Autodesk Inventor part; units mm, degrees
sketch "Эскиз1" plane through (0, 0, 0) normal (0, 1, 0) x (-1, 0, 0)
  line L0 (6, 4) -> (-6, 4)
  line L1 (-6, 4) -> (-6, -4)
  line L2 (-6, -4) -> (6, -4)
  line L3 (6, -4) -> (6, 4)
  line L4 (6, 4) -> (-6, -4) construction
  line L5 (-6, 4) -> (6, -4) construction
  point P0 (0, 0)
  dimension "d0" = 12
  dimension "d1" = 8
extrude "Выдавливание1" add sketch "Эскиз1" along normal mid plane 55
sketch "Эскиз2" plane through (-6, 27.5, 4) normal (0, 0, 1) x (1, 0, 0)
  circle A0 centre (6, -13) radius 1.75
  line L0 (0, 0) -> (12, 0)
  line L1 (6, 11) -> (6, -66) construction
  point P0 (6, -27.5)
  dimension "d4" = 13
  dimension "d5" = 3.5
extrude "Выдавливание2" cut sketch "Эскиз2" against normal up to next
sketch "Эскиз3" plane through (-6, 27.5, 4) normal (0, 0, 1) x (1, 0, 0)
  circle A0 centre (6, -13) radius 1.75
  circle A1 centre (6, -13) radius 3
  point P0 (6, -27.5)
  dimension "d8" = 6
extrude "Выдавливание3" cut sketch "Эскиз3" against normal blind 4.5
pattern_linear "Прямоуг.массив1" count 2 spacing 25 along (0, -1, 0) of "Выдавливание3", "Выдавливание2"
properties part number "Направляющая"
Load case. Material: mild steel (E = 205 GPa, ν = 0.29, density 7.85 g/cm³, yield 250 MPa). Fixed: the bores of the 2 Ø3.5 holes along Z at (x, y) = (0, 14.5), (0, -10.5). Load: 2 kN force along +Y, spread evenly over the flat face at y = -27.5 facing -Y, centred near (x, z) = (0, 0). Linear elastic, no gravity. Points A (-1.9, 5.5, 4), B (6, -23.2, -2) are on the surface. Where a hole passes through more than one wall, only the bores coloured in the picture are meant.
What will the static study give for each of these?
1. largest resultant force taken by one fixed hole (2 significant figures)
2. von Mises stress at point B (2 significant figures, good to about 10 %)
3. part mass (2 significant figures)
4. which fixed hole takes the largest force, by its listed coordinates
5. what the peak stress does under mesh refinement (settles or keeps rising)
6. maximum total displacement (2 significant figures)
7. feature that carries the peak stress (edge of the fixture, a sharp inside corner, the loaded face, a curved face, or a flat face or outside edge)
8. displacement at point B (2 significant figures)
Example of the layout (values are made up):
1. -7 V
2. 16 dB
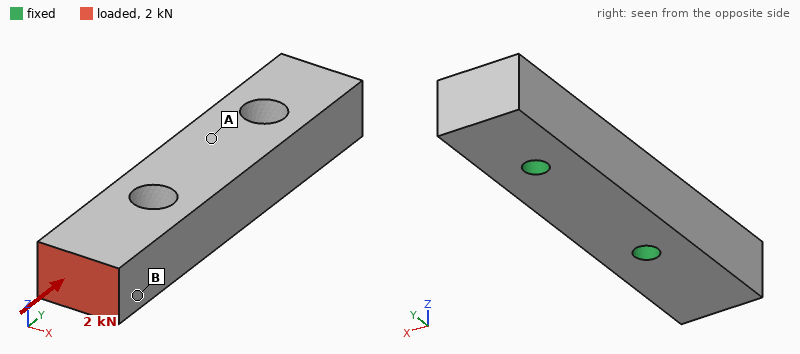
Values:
1. 1.6 kN
2. 21 MPa
3. 39 g
4. (0, -10.5)
5. keeps rising
6. 6.2 µm
7. edge of the fixture
8. 3.8 µm
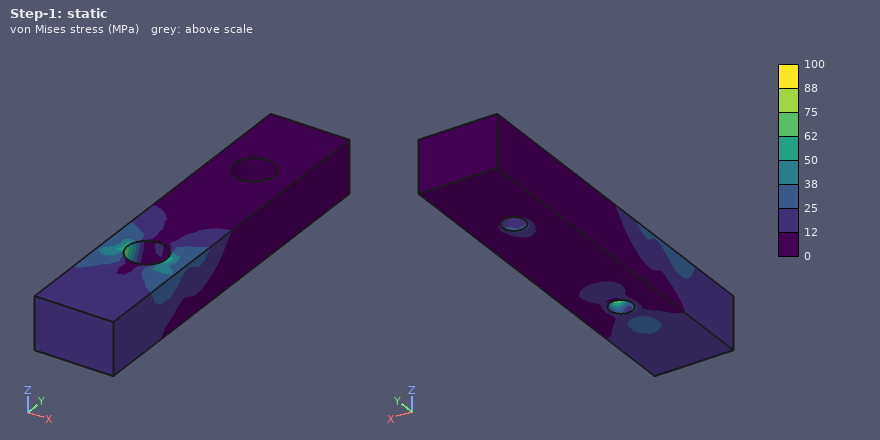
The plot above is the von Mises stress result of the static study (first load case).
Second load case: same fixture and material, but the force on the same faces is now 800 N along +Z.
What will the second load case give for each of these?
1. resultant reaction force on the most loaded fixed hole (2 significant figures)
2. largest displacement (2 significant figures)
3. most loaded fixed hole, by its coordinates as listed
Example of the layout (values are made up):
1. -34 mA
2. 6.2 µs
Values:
1. 1.4 kN
2. 28 µm
3. (0, -10.5)
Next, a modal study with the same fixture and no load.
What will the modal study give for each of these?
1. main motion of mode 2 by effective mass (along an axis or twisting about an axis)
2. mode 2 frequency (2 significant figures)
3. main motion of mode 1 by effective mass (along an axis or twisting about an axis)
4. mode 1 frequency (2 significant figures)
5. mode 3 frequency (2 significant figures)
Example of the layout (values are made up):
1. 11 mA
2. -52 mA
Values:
1. along X
2. 17 kHz
3. along Z
4. 14 kHz
5. 21 kHz
